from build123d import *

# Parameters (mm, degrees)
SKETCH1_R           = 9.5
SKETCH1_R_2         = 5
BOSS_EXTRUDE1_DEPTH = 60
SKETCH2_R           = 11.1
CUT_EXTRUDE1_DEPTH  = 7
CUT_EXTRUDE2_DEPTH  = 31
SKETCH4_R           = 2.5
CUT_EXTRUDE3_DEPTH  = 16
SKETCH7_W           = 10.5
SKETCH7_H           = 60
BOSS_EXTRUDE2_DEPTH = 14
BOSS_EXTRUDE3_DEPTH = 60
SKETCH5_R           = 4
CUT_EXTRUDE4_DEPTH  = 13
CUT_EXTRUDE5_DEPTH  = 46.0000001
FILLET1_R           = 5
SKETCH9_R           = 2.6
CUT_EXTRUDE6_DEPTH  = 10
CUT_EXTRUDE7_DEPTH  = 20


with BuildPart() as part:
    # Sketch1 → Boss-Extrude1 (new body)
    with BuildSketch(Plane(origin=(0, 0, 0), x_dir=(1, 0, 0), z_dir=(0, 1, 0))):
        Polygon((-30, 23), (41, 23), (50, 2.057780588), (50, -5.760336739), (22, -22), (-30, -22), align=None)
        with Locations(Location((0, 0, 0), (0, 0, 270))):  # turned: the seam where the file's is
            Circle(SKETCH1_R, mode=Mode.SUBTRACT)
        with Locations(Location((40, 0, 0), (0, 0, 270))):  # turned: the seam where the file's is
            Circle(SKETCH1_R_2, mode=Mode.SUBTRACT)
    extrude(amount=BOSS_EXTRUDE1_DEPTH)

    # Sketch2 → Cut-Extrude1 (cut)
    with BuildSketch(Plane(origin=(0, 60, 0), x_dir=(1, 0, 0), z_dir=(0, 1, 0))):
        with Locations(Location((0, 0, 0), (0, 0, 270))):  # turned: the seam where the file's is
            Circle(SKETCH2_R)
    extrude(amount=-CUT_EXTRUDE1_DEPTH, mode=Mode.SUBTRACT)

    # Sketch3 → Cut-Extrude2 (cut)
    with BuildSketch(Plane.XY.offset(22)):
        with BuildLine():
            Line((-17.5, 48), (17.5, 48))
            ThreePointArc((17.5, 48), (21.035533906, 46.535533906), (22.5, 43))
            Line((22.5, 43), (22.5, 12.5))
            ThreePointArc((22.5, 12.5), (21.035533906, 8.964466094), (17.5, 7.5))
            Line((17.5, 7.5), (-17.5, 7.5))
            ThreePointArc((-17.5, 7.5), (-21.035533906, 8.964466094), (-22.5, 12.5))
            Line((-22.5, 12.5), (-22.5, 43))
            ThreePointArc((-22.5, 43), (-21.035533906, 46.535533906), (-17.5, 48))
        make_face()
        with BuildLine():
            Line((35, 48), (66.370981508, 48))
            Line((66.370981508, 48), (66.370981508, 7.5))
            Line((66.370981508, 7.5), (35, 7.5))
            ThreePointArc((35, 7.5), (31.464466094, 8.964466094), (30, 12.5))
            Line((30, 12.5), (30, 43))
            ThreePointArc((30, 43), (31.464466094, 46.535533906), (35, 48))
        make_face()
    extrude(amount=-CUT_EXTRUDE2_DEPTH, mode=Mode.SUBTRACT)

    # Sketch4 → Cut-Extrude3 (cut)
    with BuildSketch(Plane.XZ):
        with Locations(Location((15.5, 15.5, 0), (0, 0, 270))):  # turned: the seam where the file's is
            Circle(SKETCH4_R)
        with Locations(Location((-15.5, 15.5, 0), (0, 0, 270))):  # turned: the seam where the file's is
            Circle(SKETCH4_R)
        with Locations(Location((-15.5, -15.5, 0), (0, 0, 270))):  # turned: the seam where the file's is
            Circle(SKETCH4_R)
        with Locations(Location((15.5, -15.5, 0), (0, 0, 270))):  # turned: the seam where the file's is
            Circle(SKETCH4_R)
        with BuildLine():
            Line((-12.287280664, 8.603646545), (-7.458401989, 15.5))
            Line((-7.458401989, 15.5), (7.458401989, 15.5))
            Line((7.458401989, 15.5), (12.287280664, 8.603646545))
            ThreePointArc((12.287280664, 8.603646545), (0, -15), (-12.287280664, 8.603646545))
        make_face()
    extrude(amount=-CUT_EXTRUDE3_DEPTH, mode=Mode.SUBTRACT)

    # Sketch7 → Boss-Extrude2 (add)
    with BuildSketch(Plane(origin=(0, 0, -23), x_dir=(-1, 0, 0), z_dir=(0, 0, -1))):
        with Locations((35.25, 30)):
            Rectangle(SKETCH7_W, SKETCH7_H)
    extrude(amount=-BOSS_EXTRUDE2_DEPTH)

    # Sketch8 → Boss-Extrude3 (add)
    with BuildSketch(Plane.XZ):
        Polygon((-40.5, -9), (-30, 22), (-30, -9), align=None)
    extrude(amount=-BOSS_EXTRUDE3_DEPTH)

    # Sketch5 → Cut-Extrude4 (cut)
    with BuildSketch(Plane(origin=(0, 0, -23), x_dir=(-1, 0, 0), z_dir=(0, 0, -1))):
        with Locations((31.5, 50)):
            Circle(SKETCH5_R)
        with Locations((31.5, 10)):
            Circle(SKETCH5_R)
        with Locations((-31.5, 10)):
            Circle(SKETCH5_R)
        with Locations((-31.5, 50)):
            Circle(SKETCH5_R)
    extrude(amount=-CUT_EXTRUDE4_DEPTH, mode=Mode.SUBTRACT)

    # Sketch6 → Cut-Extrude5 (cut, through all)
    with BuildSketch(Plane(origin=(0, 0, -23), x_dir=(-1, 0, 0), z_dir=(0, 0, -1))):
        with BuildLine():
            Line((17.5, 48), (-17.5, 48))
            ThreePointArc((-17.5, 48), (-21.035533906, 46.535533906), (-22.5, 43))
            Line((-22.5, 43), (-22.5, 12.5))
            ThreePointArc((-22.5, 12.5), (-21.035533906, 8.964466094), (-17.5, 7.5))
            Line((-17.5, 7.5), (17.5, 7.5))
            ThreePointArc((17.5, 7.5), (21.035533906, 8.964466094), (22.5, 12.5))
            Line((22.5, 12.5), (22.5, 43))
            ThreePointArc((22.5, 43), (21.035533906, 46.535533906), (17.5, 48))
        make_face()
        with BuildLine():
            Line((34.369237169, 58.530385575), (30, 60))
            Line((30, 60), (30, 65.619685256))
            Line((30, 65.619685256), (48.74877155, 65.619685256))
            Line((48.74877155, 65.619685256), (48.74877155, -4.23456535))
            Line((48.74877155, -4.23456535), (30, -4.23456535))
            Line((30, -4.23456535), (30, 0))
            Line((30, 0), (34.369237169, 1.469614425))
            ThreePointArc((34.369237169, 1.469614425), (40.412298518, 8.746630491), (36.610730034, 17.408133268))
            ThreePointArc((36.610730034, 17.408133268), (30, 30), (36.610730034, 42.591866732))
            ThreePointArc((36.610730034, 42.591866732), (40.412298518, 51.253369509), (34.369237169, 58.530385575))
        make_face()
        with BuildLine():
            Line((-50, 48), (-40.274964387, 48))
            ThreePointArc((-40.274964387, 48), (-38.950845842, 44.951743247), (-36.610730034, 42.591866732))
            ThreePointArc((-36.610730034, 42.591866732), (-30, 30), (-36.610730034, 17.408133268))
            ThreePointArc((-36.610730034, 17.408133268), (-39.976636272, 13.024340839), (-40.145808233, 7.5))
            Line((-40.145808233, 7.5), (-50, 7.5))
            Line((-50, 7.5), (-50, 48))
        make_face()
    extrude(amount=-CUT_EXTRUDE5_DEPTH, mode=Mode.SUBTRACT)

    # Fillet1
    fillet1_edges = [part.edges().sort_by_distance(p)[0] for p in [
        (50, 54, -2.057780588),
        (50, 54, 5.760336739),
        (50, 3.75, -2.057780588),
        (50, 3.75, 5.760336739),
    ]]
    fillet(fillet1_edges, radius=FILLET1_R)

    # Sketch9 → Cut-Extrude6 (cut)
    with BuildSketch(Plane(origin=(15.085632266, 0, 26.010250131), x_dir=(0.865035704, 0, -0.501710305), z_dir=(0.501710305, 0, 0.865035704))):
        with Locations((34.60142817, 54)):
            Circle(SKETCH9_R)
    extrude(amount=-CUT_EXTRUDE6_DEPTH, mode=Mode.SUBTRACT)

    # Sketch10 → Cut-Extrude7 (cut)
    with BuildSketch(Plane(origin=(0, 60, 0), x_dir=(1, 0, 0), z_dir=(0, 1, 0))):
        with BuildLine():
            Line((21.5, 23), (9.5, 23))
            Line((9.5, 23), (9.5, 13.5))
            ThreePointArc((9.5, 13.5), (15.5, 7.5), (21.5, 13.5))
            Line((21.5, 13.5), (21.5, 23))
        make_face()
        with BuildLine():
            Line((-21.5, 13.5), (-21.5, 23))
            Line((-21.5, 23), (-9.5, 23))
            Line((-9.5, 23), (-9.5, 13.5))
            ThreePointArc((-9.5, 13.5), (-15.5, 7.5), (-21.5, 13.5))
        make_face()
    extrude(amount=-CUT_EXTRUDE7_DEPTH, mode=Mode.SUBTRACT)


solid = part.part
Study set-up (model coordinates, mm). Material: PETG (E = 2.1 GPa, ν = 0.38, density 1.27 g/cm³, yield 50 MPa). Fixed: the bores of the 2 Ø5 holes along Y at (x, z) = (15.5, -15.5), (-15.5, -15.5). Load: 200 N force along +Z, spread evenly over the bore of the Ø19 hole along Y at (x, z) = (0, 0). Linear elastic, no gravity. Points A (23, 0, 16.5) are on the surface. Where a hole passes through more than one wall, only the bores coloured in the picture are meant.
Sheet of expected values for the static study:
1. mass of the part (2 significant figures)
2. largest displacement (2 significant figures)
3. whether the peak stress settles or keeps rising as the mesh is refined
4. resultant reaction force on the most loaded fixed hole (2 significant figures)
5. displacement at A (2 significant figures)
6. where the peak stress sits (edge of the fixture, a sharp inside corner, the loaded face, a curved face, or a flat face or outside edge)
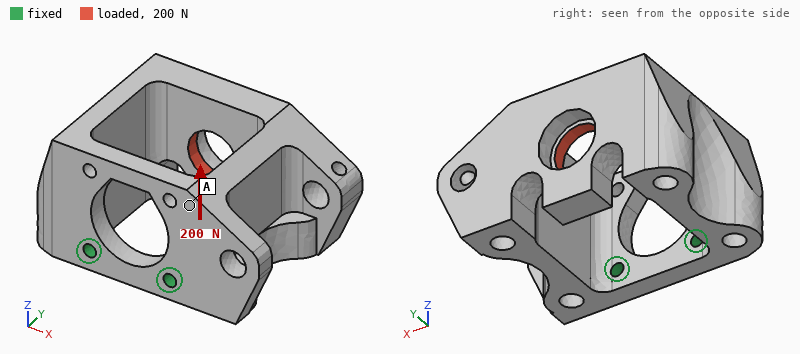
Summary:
110 g
1.4 mm
keeps rising
100 N
0.62 mm
edge of the fixture
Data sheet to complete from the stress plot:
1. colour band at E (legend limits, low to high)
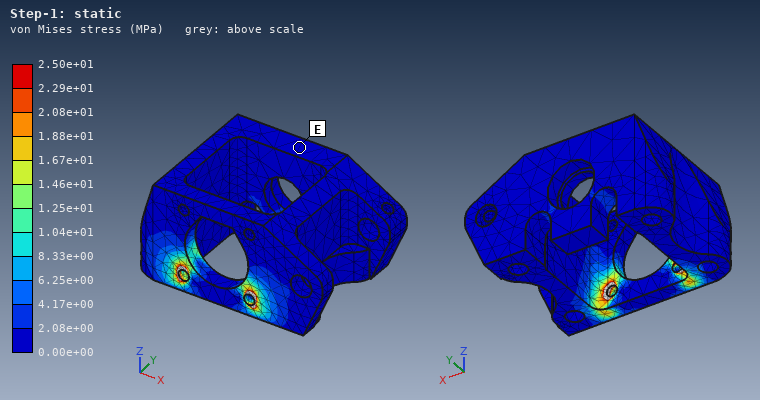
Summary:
0.00e+00 to 2.08e+00 MPa
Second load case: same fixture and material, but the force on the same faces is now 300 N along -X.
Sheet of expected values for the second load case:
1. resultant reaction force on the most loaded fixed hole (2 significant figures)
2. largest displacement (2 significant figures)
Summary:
270 N
1.2 mm
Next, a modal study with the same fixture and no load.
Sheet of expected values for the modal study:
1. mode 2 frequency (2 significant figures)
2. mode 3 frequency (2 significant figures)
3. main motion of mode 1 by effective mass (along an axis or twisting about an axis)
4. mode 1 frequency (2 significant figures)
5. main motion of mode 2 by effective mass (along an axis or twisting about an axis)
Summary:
340 Hz
560 Hz
along Z
260 Hz
along X
